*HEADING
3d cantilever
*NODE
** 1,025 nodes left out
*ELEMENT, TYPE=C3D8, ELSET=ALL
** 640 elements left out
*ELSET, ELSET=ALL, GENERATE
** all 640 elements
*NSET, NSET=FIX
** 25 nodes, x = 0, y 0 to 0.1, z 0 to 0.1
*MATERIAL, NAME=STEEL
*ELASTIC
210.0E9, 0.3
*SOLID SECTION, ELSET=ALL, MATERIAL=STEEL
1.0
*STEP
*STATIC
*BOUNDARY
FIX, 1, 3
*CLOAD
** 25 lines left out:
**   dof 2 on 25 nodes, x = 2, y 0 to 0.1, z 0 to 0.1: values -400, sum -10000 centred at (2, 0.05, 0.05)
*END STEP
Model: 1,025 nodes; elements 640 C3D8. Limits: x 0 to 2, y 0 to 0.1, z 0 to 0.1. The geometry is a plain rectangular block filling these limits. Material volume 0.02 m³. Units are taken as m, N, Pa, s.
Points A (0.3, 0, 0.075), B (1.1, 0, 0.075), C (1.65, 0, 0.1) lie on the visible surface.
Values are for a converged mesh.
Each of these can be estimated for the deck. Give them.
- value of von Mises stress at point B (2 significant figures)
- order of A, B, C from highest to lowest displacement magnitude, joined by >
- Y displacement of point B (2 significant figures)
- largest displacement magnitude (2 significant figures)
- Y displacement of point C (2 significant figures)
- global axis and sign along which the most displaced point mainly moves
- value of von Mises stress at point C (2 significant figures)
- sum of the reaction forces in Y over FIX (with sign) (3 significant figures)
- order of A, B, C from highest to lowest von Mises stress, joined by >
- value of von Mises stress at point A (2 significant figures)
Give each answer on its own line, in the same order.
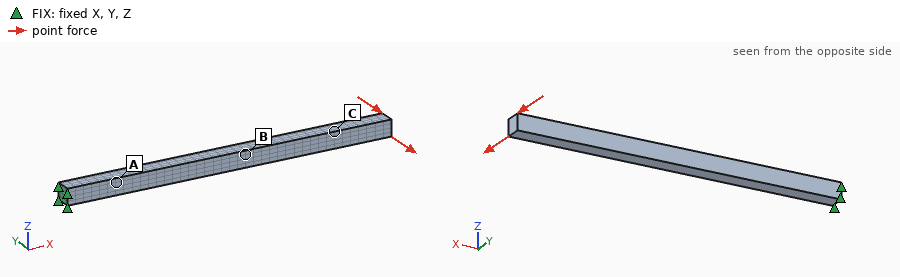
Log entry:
5.4e+07 Pa
C > B > A
-0.0056 m
0.015 m
-0.011 m
-Y
2.1e+07 Pa
10000 N
A > B > C
1.0e+08 Pa
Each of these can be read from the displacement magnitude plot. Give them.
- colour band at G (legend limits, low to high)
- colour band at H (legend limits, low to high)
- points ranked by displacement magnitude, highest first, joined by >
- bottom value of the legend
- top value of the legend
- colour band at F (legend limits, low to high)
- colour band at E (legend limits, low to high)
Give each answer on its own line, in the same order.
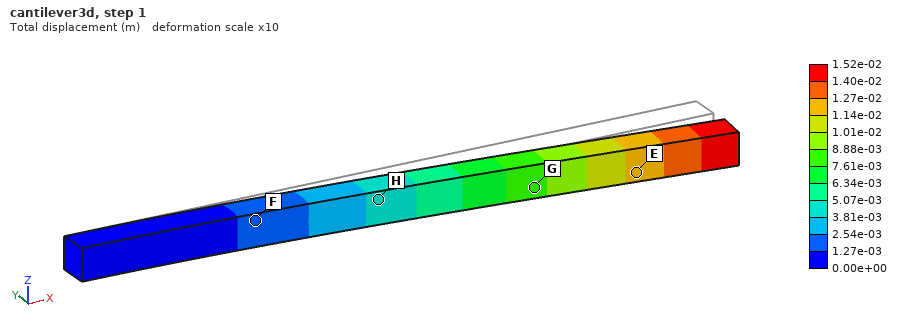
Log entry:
7.61e-03 to 8.88e-03 m
3.81e-03 to 5.07e-03 m
E > G > H > F
0.00e+00 m
1.52e-02 m
1.27e-03 to 2.54e-03 m
1.14e-02 to 1.27e-02 m
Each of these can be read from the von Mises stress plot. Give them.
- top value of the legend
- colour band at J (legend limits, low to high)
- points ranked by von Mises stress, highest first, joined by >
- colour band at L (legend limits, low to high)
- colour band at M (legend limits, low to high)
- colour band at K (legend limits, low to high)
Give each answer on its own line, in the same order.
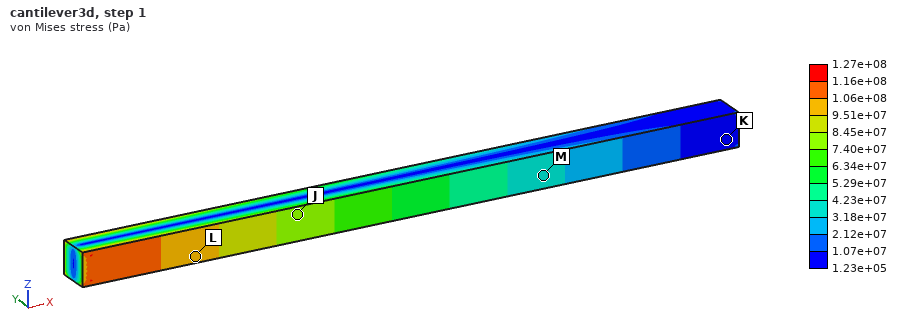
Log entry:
1.27e+08 Pa
7.40e+07 to 8.45e+07 Pa
L > J > M > K
9.51e+07 to 1.06e+08 Pa
3.18e+07 to 4.23e+07 Pa
1.23e+05 to 1.07e+07 Pa
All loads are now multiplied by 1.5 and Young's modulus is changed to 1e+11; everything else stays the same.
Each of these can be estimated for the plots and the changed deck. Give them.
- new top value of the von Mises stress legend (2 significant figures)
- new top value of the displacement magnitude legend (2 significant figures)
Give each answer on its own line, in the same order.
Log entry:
1.9e+08 Pa
0.048 m
